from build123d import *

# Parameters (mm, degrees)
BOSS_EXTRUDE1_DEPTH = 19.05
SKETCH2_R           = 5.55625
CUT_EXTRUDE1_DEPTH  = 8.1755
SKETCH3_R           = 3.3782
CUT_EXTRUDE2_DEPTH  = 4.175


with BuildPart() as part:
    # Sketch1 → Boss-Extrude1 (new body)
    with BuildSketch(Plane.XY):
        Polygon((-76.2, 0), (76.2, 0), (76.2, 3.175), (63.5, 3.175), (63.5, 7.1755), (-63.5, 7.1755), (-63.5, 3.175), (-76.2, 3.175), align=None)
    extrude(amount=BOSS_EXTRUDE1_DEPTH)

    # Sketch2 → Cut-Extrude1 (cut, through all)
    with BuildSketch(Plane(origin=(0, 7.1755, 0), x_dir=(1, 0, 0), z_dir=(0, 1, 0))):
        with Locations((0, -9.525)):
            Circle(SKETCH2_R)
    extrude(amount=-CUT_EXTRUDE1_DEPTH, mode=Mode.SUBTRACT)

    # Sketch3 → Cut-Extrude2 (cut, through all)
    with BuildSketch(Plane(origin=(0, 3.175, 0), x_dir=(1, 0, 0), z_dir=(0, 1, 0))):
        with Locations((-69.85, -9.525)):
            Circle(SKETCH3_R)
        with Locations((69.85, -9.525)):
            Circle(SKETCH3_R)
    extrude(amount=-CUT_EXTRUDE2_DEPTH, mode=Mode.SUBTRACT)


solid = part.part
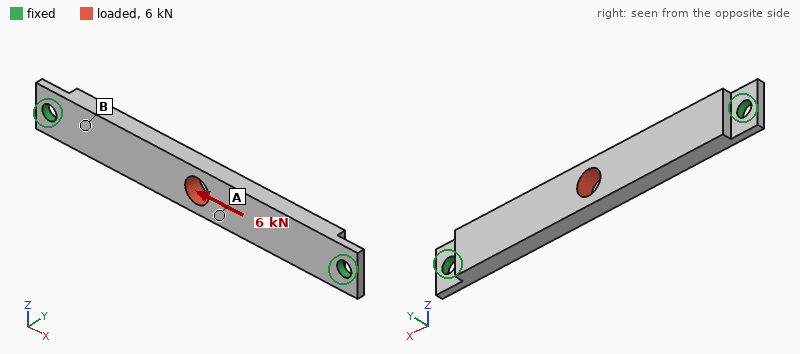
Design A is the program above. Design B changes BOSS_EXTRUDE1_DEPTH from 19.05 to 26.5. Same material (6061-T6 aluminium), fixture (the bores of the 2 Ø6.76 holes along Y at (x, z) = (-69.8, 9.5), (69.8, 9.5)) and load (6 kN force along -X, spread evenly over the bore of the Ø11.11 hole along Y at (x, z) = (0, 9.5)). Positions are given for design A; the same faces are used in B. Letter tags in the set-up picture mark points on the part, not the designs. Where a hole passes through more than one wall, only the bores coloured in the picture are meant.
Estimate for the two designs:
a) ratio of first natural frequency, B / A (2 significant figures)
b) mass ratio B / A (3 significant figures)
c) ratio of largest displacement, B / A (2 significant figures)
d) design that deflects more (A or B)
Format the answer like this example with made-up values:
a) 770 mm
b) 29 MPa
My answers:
a) 0.96
b) 1.41
c) 0.88
d) A
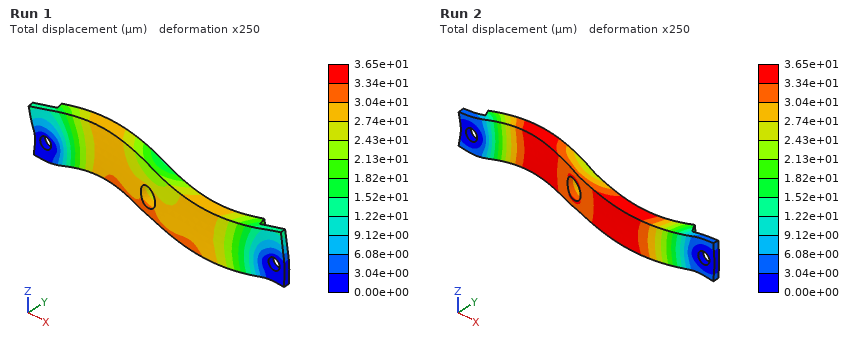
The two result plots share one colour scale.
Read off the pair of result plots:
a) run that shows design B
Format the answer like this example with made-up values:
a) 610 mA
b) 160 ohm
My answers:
a) Run 1
